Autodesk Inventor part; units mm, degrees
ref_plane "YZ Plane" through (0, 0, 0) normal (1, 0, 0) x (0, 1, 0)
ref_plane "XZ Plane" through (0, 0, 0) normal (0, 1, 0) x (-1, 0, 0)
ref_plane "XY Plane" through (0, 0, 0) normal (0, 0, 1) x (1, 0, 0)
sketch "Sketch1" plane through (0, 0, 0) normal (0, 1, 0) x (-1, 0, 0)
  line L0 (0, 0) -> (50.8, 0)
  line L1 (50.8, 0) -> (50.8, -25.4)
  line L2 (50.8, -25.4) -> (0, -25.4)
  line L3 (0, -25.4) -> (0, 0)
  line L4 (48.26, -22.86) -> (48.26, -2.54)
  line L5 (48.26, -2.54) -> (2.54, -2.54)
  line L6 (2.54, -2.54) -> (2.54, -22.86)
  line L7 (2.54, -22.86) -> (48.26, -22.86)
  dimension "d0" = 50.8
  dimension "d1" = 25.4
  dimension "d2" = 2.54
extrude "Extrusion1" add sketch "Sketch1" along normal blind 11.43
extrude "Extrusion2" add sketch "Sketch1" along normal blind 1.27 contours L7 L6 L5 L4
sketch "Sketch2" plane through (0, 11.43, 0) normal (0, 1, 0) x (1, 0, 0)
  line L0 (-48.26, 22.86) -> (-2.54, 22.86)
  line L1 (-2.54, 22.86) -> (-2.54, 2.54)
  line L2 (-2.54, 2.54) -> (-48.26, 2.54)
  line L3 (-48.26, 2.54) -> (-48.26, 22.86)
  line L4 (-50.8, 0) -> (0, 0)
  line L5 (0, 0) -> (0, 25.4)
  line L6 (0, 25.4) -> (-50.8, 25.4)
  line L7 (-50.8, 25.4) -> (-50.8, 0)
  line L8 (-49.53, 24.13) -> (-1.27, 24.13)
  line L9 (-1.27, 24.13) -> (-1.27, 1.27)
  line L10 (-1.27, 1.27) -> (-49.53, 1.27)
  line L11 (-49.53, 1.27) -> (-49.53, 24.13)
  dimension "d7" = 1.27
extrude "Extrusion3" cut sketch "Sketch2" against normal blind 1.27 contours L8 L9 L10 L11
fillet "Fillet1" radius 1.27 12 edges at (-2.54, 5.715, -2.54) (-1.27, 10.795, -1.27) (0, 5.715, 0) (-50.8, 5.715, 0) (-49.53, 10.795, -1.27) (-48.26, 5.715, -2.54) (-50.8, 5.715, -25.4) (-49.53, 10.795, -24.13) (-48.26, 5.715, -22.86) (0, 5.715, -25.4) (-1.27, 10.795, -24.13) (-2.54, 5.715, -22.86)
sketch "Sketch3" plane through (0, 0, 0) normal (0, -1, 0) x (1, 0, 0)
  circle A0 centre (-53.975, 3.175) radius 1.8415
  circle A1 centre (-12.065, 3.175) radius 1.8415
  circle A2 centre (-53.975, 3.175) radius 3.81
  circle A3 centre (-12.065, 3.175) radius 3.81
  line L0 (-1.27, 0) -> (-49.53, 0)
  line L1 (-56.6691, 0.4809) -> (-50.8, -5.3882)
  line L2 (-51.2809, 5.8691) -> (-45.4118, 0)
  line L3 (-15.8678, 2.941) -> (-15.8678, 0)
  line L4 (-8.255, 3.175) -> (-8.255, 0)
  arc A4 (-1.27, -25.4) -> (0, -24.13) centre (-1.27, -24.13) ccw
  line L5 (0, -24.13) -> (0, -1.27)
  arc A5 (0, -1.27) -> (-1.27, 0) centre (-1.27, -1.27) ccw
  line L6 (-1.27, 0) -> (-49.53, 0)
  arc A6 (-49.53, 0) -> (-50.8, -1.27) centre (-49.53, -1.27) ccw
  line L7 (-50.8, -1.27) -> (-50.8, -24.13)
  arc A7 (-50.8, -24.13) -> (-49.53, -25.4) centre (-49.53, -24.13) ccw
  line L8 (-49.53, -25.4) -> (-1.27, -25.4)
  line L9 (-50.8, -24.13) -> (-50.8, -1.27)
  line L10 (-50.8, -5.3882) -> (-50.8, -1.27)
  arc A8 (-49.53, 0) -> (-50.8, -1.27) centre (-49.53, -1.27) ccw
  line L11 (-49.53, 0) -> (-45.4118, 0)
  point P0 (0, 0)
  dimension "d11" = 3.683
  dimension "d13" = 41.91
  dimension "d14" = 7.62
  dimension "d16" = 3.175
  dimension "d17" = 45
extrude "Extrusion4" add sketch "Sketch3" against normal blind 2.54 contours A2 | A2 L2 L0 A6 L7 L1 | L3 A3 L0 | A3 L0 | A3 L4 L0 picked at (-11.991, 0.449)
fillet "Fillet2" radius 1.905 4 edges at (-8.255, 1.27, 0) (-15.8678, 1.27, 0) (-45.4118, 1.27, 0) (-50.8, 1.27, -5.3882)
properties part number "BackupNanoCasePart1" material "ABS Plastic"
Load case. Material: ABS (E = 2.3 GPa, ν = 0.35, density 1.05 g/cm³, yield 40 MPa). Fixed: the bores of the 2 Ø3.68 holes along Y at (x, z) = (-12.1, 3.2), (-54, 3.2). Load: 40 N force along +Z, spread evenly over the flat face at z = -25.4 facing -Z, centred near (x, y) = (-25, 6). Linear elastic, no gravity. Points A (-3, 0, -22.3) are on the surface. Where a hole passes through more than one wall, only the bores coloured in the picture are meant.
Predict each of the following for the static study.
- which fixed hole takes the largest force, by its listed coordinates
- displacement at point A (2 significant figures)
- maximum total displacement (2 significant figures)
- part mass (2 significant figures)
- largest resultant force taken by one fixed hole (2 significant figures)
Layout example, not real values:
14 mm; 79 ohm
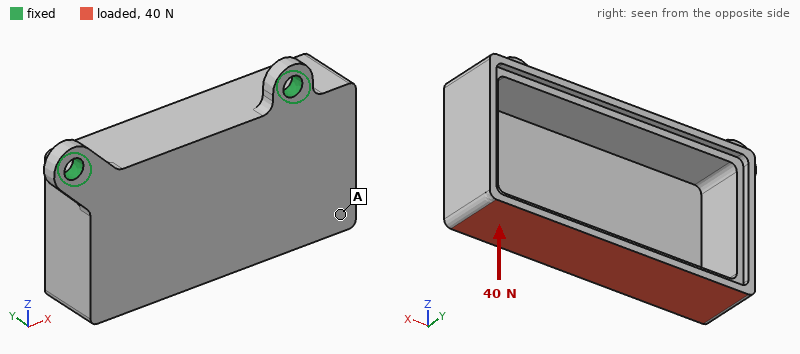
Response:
(-12.1, 3.2); 0.45 mm; 0.65 mm; 5.6 g; 26 N
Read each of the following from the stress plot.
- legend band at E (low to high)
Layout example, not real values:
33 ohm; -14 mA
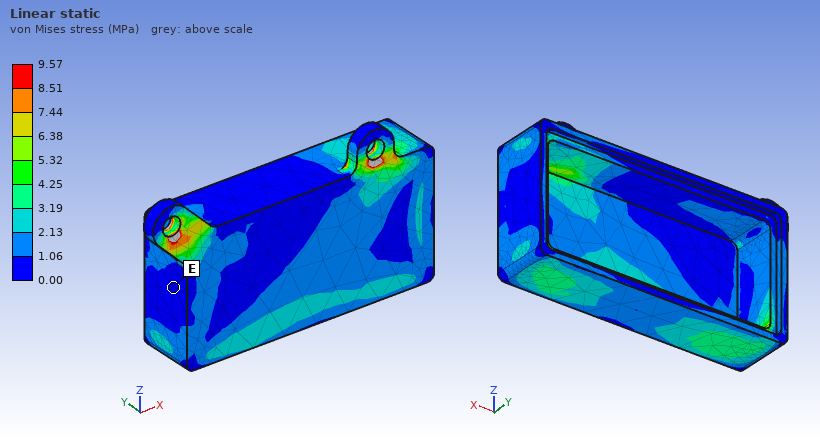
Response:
0.00 to 1.06 MPa
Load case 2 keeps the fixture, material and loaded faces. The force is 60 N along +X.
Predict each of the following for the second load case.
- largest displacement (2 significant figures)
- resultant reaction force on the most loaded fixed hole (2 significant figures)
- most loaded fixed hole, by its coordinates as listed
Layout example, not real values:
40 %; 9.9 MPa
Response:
0.45 mm; 54 N; (-54, 3.2)
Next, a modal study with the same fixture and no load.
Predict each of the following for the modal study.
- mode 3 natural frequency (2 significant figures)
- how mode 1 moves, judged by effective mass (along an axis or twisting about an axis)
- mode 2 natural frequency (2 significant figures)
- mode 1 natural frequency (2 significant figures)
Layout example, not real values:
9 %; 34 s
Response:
2500 Hz; along Y; 860 Hz; 410 Hz
